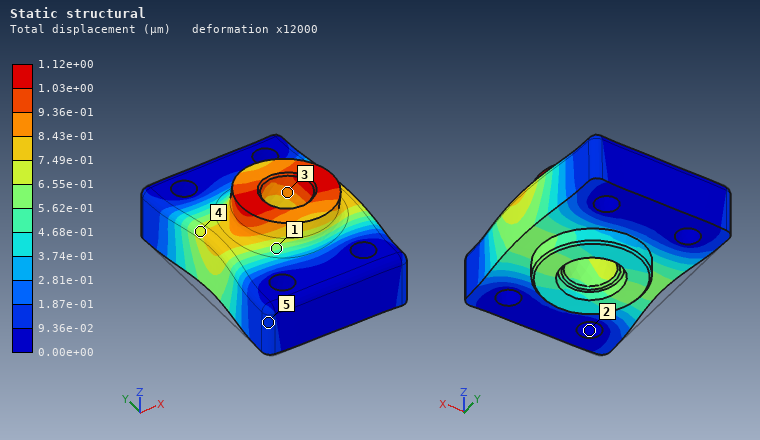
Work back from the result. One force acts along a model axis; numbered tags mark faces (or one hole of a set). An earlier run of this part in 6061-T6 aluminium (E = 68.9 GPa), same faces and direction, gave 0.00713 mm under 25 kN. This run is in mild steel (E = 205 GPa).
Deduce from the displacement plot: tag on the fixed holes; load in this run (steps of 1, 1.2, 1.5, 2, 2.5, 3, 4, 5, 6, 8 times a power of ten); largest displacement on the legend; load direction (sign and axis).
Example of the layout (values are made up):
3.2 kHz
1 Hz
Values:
2
12 kN
1.12e+00 µm
+X
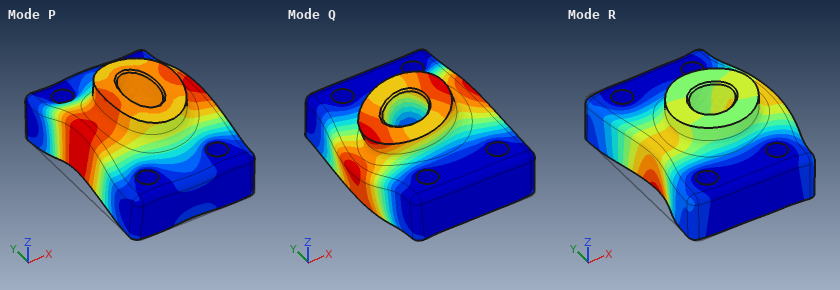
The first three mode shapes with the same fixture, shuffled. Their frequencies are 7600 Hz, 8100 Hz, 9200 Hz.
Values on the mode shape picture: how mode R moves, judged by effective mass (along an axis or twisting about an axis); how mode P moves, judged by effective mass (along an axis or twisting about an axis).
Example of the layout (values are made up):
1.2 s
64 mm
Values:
along X
along Z
